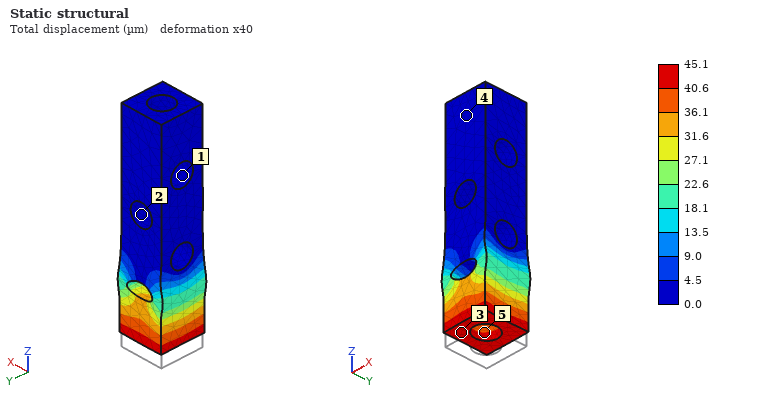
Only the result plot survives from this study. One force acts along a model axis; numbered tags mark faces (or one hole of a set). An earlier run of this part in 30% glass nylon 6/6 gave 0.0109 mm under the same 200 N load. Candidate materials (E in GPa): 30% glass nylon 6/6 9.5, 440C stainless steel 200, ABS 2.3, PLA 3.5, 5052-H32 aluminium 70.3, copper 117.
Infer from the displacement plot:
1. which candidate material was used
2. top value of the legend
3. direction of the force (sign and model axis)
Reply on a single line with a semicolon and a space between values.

ABS; 45.1 µm; +Z
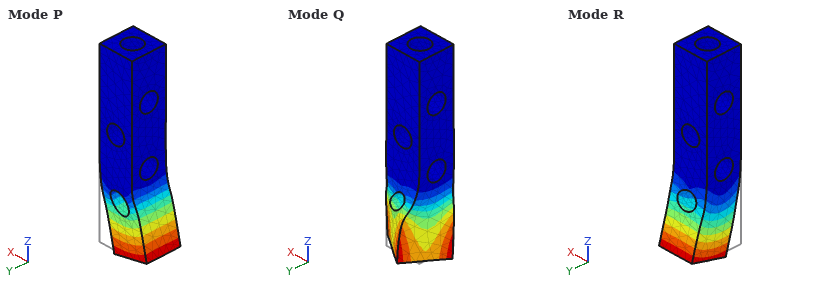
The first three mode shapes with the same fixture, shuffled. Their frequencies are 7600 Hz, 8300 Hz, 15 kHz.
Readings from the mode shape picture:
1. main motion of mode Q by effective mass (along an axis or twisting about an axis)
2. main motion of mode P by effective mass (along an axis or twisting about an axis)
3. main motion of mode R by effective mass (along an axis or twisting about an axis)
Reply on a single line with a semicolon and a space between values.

twisting about Z; along X; along Y
